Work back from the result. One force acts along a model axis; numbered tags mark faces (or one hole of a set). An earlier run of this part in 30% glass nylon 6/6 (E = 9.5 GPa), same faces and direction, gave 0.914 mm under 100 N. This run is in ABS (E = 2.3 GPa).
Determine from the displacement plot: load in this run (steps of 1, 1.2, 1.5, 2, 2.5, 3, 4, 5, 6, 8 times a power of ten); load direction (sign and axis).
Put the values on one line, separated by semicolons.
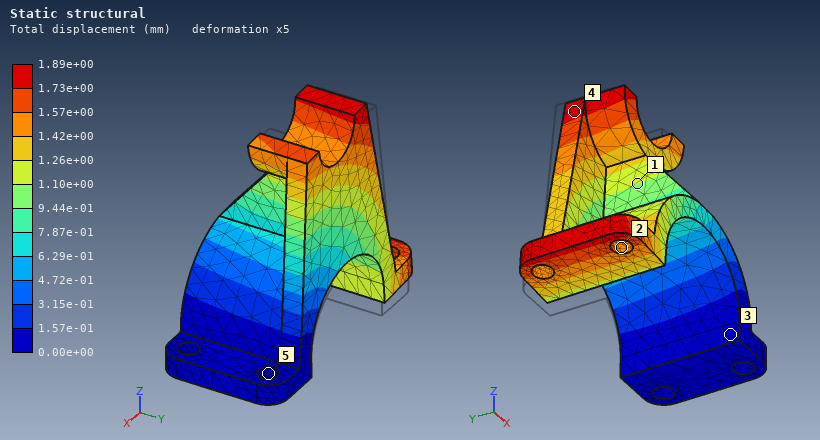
50 N; +Z
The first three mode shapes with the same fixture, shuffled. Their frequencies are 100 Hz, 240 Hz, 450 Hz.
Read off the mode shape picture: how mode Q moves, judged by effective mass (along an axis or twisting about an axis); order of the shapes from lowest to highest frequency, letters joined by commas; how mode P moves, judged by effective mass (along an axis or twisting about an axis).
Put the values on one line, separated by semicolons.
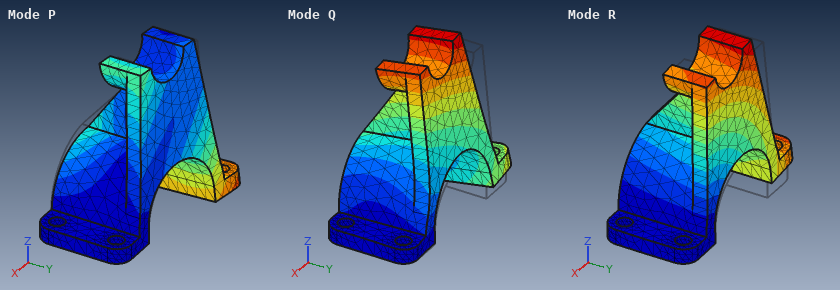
along Y; R, P, Q; along Y
